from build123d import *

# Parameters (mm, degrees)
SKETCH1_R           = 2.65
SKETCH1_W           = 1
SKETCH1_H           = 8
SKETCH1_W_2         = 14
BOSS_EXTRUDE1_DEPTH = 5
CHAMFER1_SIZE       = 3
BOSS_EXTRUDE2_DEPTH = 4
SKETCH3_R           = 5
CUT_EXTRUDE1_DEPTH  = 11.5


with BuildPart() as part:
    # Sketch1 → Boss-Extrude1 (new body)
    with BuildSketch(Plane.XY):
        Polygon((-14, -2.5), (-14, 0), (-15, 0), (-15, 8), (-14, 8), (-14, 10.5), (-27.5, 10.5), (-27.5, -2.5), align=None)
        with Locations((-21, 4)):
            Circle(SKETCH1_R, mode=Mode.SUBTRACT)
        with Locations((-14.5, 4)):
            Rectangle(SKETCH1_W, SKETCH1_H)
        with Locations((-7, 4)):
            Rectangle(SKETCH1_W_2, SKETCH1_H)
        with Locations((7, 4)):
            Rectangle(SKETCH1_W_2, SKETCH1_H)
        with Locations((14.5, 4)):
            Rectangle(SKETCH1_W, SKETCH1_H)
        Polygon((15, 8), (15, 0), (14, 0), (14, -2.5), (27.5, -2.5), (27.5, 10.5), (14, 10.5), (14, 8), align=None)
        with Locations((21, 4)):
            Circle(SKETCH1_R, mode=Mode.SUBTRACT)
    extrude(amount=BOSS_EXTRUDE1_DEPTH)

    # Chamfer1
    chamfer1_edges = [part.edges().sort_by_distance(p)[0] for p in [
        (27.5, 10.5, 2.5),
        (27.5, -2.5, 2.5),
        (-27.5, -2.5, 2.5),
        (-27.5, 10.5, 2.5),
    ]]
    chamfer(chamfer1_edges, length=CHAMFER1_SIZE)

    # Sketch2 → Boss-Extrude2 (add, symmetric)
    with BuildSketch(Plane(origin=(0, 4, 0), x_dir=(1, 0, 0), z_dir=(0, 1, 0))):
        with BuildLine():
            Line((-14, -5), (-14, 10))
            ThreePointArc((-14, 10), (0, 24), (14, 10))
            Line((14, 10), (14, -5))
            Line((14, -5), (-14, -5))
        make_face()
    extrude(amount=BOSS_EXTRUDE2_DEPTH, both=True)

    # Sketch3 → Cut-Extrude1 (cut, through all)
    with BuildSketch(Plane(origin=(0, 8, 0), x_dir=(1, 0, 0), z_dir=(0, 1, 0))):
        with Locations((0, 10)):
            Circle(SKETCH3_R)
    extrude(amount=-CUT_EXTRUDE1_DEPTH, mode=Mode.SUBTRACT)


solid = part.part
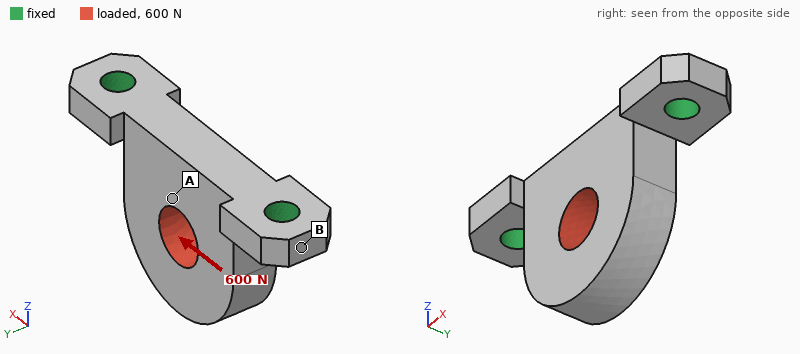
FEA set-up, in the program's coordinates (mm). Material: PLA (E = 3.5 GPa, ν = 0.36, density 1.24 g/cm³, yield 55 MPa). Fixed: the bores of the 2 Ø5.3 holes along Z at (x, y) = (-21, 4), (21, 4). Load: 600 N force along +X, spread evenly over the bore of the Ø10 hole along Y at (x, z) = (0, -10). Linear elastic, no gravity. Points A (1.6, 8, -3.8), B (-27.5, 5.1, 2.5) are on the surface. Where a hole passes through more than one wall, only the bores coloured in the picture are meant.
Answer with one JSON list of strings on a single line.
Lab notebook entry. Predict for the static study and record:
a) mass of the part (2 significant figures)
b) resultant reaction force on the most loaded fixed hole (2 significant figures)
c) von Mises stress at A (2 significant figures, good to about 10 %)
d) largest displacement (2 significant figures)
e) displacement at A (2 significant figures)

["8.2 g", "380 N", "7.3 MPa", "0.14 mm", "0.043 mm"]
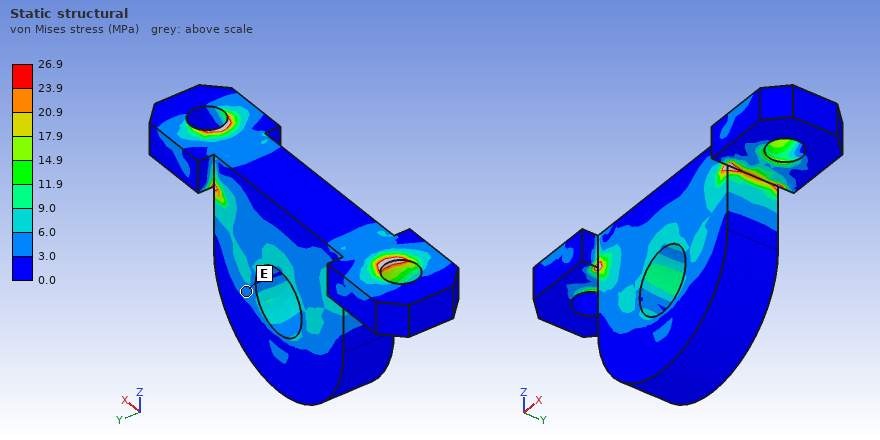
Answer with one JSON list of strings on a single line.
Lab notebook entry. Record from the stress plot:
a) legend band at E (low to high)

["3.0 to 6.0 MPa"]
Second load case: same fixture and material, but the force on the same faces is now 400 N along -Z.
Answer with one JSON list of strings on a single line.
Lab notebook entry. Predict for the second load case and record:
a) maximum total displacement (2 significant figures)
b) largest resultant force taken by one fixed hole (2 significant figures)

["67 µm", "230 N"]
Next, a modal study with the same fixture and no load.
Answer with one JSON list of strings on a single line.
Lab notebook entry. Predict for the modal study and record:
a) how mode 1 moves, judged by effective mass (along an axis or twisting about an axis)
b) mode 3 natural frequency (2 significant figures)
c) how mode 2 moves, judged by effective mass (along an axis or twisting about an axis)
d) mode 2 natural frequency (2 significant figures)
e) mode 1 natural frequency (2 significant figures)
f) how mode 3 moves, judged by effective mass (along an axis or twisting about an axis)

["along Y", "5200 Hz", "along X", "4900 Hz", "1500 Hz", "along Z"]
